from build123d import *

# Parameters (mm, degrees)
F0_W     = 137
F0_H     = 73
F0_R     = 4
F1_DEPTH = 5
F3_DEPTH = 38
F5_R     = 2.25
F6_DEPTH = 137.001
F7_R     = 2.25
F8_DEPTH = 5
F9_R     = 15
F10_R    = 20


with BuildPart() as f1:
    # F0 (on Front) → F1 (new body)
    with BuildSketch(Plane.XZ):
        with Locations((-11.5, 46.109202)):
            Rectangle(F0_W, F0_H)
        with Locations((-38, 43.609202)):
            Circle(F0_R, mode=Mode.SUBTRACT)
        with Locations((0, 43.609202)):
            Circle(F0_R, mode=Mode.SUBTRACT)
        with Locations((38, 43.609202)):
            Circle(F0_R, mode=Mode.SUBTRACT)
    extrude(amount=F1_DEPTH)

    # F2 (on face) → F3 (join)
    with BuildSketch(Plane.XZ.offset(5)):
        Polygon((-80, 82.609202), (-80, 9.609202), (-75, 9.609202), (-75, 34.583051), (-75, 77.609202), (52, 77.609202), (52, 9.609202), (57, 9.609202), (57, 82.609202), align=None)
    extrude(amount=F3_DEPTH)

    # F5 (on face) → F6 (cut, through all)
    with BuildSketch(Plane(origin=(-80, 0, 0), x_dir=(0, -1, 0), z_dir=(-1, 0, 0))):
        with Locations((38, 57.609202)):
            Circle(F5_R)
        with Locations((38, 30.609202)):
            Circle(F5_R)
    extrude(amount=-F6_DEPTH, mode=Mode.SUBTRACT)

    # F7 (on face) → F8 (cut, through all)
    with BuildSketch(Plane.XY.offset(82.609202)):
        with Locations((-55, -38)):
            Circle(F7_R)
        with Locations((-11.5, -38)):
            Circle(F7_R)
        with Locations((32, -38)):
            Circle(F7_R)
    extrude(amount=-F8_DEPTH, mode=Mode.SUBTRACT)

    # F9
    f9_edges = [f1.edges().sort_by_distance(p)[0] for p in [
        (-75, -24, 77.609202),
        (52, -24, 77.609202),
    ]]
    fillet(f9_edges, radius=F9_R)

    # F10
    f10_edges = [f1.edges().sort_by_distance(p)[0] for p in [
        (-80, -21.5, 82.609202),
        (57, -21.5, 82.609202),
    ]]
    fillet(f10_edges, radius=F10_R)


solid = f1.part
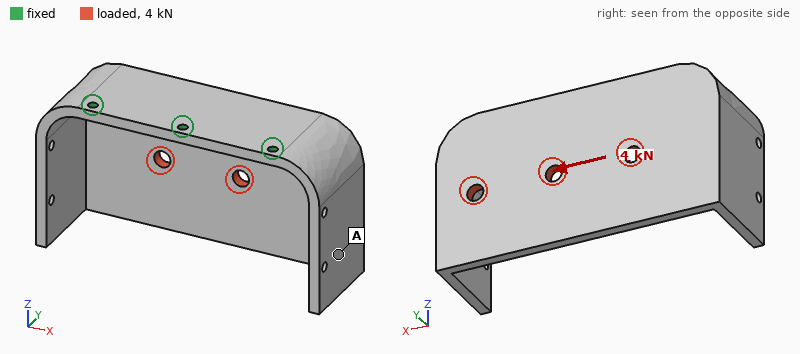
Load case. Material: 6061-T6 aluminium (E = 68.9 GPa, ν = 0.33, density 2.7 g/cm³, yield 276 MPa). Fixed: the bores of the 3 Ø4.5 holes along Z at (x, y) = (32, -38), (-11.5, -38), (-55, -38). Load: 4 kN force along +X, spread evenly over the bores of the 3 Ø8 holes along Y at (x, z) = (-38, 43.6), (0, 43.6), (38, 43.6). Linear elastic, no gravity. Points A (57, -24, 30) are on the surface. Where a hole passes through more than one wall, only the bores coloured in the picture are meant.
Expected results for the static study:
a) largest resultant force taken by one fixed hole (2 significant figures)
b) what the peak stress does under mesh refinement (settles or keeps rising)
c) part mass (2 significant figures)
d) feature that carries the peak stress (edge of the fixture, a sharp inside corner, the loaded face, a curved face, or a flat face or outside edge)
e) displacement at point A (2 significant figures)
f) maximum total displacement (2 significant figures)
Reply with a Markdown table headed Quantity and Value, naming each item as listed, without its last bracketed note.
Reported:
| Quantity | Value |
|---|---|
| largest resultant force taken by one fixed hole | 2.5 kN |
| what the peak stress does under mesh refinement | keeps rising |
| part mass | 260 g |
| feature that carries the peak stress | edge of the fixture |
| displacement at point A | 0.73 mm |
| maximum total displacement | 1.0 mm |
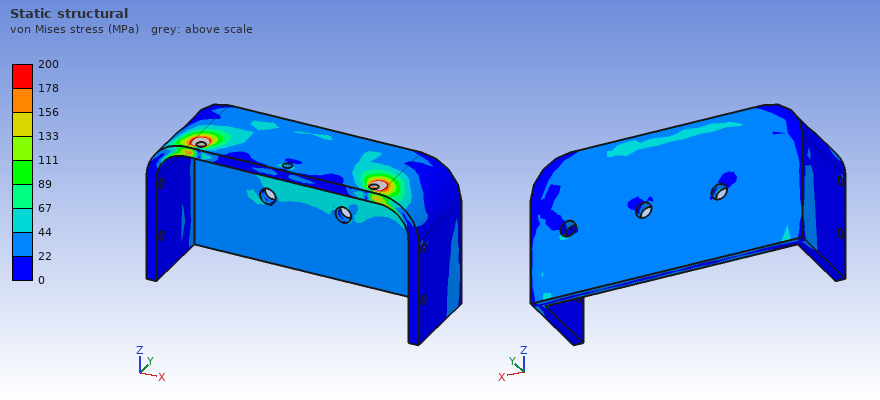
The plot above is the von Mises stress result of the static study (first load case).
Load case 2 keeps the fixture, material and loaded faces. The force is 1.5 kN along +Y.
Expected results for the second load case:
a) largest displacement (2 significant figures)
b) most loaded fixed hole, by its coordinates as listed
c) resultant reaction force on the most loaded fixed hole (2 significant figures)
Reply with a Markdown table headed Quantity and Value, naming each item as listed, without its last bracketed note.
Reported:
| Quantity | Value |
|---|---|
| largest displacement | 1.2 mm |
| most loaded fixed hole, by its coordinates as listed | (32, -38) |
| resultant reaction force on the most loaded fixed hole | 750 N |
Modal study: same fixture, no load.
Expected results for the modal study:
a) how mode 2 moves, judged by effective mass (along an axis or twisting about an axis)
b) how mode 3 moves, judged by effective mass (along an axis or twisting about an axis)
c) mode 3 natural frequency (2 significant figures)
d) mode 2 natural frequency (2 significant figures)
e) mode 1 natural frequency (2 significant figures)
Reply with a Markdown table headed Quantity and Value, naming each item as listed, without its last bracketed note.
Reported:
| Quantity | Value |
|---|---|
| how mode 2 moves, judged by effective mass | along X |
| how mode 3 moves, judged by effective mass | along Z |
| mode 3 natural frequency | 1600 Hz |
| mode 2 natural frequency | 670 Hz |
| mode 1 natural frequency | 500 Hz |
